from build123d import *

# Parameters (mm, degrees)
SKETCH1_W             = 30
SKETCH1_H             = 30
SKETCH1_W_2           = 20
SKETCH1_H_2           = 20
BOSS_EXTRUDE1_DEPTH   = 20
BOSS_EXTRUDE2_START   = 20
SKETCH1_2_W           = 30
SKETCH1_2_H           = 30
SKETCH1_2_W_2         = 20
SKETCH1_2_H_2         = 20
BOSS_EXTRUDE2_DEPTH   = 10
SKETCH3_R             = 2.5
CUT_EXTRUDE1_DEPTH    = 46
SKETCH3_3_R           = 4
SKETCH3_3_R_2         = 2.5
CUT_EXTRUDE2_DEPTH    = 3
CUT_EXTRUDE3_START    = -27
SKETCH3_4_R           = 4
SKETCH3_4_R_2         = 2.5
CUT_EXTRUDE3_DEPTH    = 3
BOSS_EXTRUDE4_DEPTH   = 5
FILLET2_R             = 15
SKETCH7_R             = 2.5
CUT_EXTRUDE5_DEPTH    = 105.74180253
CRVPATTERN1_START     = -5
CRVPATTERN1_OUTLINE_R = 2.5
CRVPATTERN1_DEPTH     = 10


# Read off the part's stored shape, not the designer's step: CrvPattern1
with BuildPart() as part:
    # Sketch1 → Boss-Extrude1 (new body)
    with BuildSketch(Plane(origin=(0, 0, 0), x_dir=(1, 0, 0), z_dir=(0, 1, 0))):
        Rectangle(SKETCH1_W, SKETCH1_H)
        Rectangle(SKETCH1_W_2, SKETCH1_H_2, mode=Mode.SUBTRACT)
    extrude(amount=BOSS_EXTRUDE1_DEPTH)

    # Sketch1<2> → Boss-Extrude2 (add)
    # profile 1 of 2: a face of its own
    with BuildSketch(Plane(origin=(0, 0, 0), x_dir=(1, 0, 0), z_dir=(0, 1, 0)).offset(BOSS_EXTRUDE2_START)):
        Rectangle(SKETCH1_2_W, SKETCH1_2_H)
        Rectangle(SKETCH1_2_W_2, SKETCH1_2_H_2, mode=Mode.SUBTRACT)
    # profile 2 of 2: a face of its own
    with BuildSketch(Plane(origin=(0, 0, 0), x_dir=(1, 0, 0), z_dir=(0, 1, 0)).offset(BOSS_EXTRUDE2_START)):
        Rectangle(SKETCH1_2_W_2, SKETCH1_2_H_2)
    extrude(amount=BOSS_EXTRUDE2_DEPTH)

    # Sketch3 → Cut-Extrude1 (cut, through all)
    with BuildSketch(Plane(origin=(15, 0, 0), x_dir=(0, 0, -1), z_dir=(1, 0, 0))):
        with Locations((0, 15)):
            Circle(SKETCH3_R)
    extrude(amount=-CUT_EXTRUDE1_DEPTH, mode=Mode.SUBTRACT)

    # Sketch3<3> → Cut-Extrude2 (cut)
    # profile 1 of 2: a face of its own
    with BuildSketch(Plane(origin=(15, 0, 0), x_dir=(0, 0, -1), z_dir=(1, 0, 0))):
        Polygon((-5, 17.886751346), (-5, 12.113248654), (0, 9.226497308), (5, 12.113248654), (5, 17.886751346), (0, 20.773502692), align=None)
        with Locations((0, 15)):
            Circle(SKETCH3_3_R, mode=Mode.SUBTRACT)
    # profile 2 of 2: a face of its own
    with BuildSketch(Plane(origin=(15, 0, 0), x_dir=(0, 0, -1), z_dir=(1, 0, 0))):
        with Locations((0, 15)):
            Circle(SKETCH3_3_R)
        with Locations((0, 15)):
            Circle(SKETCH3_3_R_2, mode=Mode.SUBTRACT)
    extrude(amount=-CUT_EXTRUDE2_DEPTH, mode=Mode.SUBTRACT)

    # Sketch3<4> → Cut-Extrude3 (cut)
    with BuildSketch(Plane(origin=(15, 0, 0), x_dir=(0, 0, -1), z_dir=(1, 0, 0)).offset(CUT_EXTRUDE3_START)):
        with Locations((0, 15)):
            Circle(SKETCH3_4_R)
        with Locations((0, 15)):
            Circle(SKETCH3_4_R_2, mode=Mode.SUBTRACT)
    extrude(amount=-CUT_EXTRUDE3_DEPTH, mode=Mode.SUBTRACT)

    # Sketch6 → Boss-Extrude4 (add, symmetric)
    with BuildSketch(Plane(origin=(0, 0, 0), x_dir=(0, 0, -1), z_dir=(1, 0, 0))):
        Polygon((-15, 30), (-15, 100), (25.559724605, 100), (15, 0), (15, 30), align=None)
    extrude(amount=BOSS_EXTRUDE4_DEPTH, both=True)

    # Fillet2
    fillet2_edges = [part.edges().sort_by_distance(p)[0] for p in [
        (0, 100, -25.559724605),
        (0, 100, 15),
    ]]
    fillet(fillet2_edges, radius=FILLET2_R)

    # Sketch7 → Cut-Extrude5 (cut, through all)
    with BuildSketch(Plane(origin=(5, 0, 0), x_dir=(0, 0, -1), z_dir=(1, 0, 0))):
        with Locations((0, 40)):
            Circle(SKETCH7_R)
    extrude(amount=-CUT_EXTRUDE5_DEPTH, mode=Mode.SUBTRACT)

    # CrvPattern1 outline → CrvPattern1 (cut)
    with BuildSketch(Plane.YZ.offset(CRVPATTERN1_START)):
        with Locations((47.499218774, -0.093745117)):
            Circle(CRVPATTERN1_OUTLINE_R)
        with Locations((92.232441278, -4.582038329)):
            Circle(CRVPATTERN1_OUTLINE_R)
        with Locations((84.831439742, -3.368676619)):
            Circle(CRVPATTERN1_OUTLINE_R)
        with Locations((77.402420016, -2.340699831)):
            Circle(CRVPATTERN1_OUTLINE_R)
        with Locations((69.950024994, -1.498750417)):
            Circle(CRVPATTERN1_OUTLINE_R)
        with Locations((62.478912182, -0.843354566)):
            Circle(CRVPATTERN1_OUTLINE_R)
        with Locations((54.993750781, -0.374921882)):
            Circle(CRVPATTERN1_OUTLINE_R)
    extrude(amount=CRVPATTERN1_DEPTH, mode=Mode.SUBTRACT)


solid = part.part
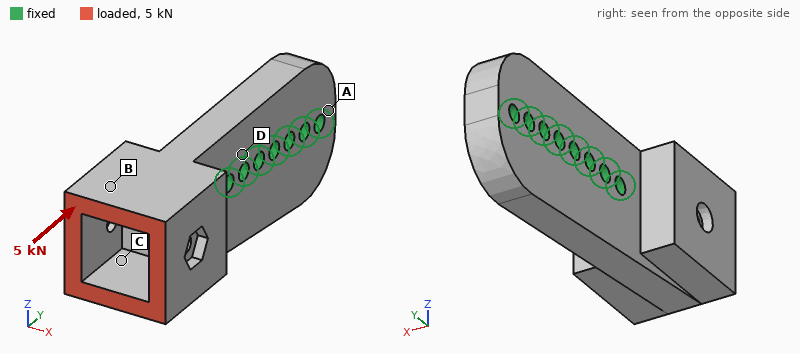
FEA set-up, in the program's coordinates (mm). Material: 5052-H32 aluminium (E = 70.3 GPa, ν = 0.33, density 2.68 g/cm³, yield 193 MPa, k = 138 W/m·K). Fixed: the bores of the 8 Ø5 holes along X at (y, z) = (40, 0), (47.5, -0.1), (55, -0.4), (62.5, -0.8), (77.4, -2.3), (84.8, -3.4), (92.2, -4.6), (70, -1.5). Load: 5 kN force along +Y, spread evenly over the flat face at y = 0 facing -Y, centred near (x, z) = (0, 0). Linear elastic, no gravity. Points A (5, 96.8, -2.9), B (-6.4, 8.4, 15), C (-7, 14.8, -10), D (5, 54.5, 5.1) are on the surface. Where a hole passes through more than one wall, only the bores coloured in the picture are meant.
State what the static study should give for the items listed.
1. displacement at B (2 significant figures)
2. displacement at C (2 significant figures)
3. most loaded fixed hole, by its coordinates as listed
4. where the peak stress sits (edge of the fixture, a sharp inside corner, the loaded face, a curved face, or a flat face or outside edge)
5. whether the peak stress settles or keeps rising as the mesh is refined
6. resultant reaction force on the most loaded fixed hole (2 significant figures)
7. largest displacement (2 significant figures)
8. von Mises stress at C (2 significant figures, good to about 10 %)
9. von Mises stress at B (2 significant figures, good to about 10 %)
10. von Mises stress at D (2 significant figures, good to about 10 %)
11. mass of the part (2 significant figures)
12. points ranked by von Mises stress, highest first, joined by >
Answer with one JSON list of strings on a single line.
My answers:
["9.8 µm", "6.4 µm", "(40, 0)", "edge of the fixture", "keeps rising", "3.1 kN", "12 µm", "14 MPa", "11 MPa", "5.3 MPa", "110 g", "C > B > D > A"]
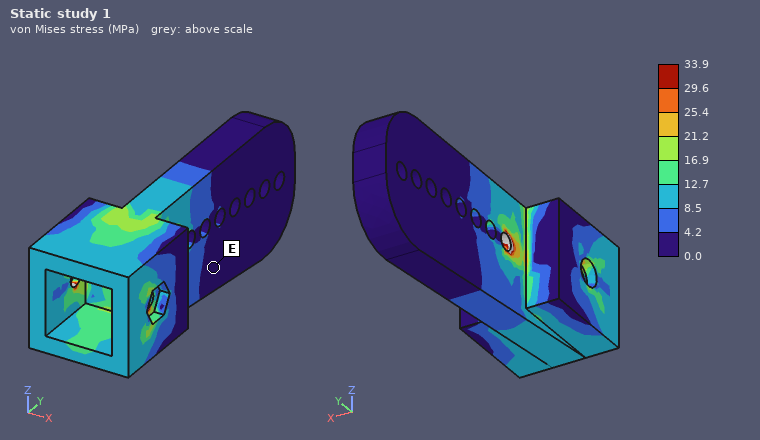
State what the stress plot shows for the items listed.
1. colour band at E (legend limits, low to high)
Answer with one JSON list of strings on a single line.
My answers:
["0.0 to 4.2 MPa"]
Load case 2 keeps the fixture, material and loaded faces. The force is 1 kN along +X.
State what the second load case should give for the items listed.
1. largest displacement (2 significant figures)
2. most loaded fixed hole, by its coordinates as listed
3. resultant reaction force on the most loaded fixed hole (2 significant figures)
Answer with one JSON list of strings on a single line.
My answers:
["0.11 mm", "(40, 0)", "2.0 kN"]
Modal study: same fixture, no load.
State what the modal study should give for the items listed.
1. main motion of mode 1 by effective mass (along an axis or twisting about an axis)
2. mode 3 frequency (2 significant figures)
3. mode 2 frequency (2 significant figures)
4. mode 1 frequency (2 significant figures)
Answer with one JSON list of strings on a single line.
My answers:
["along X", "7200 Hz", "7000 Hz", "3600 Hz"]
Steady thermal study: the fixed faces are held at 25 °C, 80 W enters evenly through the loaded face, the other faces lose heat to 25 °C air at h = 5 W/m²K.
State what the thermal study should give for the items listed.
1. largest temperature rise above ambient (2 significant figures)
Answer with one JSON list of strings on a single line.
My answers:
["60 K"]
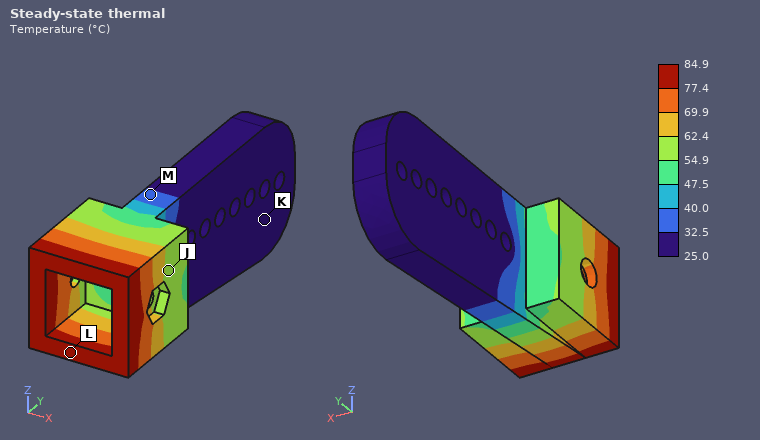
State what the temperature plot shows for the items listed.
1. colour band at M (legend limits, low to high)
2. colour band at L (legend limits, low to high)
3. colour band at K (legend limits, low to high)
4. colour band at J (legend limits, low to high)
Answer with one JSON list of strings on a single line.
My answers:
["32.5 to 40.0 °C", "77.4 to 84.9 °C", "25.0 to 32.5 °C", "54.9 to 62.4 °C"]
